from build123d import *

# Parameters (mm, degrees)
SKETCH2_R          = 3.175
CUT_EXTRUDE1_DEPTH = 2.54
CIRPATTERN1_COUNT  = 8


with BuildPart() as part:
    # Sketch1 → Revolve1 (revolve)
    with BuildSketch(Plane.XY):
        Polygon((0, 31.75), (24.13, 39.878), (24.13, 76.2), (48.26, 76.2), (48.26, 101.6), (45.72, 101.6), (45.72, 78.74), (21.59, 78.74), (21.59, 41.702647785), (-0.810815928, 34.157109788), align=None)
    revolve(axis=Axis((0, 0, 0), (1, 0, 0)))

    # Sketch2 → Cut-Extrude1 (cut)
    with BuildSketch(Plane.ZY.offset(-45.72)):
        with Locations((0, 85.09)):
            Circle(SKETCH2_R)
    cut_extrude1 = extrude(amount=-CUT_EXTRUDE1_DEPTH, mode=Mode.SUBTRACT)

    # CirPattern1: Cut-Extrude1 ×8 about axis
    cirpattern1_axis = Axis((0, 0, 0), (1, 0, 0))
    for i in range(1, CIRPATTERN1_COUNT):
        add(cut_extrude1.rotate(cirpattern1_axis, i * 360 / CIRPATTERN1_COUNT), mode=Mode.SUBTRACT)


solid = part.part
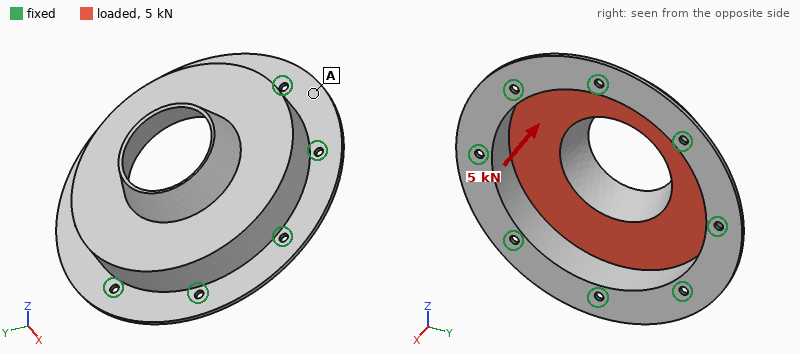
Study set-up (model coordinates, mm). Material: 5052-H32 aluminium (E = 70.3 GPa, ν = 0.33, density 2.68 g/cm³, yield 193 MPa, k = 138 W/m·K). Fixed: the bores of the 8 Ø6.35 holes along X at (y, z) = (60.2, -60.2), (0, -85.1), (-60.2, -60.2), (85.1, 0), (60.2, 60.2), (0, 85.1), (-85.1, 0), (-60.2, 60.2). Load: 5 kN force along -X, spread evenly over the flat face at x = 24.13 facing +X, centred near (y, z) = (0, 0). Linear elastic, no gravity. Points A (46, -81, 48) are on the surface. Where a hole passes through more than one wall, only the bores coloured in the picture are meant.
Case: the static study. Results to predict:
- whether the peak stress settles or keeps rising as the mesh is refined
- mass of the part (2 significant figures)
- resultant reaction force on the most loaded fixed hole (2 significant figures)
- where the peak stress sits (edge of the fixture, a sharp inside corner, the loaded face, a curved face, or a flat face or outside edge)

keeps rising
300 g
670 N
edge of the fixture
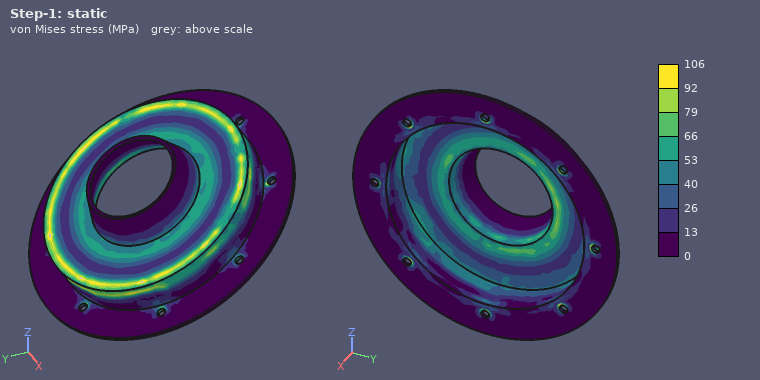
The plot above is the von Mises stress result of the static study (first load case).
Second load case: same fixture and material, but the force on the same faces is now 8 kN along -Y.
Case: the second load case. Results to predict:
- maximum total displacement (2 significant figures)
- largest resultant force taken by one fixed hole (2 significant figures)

46 µm
1.6 kN
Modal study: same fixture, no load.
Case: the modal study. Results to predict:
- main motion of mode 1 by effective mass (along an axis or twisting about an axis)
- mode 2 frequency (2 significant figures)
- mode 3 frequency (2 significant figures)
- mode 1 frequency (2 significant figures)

along X
2200 Hz
2200 Hz
1600 Hz
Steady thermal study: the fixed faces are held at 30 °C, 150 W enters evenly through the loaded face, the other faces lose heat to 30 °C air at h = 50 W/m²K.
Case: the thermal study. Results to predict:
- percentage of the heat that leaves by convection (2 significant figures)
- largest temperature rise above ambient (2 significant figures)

44 %
33 K
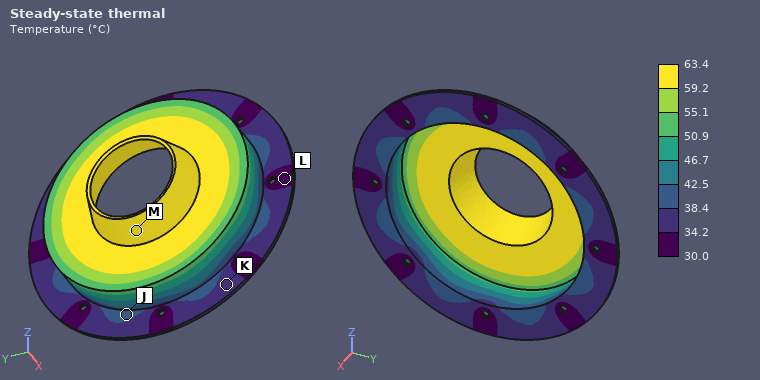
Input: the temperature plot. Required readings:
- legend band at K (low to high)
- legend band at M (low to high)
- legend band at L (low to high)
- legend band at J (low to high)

34.2 to 38.4 °C
59.2 to 63.4 °C
30.0 to 34.2 °C
38.4 to 42.5 °C
